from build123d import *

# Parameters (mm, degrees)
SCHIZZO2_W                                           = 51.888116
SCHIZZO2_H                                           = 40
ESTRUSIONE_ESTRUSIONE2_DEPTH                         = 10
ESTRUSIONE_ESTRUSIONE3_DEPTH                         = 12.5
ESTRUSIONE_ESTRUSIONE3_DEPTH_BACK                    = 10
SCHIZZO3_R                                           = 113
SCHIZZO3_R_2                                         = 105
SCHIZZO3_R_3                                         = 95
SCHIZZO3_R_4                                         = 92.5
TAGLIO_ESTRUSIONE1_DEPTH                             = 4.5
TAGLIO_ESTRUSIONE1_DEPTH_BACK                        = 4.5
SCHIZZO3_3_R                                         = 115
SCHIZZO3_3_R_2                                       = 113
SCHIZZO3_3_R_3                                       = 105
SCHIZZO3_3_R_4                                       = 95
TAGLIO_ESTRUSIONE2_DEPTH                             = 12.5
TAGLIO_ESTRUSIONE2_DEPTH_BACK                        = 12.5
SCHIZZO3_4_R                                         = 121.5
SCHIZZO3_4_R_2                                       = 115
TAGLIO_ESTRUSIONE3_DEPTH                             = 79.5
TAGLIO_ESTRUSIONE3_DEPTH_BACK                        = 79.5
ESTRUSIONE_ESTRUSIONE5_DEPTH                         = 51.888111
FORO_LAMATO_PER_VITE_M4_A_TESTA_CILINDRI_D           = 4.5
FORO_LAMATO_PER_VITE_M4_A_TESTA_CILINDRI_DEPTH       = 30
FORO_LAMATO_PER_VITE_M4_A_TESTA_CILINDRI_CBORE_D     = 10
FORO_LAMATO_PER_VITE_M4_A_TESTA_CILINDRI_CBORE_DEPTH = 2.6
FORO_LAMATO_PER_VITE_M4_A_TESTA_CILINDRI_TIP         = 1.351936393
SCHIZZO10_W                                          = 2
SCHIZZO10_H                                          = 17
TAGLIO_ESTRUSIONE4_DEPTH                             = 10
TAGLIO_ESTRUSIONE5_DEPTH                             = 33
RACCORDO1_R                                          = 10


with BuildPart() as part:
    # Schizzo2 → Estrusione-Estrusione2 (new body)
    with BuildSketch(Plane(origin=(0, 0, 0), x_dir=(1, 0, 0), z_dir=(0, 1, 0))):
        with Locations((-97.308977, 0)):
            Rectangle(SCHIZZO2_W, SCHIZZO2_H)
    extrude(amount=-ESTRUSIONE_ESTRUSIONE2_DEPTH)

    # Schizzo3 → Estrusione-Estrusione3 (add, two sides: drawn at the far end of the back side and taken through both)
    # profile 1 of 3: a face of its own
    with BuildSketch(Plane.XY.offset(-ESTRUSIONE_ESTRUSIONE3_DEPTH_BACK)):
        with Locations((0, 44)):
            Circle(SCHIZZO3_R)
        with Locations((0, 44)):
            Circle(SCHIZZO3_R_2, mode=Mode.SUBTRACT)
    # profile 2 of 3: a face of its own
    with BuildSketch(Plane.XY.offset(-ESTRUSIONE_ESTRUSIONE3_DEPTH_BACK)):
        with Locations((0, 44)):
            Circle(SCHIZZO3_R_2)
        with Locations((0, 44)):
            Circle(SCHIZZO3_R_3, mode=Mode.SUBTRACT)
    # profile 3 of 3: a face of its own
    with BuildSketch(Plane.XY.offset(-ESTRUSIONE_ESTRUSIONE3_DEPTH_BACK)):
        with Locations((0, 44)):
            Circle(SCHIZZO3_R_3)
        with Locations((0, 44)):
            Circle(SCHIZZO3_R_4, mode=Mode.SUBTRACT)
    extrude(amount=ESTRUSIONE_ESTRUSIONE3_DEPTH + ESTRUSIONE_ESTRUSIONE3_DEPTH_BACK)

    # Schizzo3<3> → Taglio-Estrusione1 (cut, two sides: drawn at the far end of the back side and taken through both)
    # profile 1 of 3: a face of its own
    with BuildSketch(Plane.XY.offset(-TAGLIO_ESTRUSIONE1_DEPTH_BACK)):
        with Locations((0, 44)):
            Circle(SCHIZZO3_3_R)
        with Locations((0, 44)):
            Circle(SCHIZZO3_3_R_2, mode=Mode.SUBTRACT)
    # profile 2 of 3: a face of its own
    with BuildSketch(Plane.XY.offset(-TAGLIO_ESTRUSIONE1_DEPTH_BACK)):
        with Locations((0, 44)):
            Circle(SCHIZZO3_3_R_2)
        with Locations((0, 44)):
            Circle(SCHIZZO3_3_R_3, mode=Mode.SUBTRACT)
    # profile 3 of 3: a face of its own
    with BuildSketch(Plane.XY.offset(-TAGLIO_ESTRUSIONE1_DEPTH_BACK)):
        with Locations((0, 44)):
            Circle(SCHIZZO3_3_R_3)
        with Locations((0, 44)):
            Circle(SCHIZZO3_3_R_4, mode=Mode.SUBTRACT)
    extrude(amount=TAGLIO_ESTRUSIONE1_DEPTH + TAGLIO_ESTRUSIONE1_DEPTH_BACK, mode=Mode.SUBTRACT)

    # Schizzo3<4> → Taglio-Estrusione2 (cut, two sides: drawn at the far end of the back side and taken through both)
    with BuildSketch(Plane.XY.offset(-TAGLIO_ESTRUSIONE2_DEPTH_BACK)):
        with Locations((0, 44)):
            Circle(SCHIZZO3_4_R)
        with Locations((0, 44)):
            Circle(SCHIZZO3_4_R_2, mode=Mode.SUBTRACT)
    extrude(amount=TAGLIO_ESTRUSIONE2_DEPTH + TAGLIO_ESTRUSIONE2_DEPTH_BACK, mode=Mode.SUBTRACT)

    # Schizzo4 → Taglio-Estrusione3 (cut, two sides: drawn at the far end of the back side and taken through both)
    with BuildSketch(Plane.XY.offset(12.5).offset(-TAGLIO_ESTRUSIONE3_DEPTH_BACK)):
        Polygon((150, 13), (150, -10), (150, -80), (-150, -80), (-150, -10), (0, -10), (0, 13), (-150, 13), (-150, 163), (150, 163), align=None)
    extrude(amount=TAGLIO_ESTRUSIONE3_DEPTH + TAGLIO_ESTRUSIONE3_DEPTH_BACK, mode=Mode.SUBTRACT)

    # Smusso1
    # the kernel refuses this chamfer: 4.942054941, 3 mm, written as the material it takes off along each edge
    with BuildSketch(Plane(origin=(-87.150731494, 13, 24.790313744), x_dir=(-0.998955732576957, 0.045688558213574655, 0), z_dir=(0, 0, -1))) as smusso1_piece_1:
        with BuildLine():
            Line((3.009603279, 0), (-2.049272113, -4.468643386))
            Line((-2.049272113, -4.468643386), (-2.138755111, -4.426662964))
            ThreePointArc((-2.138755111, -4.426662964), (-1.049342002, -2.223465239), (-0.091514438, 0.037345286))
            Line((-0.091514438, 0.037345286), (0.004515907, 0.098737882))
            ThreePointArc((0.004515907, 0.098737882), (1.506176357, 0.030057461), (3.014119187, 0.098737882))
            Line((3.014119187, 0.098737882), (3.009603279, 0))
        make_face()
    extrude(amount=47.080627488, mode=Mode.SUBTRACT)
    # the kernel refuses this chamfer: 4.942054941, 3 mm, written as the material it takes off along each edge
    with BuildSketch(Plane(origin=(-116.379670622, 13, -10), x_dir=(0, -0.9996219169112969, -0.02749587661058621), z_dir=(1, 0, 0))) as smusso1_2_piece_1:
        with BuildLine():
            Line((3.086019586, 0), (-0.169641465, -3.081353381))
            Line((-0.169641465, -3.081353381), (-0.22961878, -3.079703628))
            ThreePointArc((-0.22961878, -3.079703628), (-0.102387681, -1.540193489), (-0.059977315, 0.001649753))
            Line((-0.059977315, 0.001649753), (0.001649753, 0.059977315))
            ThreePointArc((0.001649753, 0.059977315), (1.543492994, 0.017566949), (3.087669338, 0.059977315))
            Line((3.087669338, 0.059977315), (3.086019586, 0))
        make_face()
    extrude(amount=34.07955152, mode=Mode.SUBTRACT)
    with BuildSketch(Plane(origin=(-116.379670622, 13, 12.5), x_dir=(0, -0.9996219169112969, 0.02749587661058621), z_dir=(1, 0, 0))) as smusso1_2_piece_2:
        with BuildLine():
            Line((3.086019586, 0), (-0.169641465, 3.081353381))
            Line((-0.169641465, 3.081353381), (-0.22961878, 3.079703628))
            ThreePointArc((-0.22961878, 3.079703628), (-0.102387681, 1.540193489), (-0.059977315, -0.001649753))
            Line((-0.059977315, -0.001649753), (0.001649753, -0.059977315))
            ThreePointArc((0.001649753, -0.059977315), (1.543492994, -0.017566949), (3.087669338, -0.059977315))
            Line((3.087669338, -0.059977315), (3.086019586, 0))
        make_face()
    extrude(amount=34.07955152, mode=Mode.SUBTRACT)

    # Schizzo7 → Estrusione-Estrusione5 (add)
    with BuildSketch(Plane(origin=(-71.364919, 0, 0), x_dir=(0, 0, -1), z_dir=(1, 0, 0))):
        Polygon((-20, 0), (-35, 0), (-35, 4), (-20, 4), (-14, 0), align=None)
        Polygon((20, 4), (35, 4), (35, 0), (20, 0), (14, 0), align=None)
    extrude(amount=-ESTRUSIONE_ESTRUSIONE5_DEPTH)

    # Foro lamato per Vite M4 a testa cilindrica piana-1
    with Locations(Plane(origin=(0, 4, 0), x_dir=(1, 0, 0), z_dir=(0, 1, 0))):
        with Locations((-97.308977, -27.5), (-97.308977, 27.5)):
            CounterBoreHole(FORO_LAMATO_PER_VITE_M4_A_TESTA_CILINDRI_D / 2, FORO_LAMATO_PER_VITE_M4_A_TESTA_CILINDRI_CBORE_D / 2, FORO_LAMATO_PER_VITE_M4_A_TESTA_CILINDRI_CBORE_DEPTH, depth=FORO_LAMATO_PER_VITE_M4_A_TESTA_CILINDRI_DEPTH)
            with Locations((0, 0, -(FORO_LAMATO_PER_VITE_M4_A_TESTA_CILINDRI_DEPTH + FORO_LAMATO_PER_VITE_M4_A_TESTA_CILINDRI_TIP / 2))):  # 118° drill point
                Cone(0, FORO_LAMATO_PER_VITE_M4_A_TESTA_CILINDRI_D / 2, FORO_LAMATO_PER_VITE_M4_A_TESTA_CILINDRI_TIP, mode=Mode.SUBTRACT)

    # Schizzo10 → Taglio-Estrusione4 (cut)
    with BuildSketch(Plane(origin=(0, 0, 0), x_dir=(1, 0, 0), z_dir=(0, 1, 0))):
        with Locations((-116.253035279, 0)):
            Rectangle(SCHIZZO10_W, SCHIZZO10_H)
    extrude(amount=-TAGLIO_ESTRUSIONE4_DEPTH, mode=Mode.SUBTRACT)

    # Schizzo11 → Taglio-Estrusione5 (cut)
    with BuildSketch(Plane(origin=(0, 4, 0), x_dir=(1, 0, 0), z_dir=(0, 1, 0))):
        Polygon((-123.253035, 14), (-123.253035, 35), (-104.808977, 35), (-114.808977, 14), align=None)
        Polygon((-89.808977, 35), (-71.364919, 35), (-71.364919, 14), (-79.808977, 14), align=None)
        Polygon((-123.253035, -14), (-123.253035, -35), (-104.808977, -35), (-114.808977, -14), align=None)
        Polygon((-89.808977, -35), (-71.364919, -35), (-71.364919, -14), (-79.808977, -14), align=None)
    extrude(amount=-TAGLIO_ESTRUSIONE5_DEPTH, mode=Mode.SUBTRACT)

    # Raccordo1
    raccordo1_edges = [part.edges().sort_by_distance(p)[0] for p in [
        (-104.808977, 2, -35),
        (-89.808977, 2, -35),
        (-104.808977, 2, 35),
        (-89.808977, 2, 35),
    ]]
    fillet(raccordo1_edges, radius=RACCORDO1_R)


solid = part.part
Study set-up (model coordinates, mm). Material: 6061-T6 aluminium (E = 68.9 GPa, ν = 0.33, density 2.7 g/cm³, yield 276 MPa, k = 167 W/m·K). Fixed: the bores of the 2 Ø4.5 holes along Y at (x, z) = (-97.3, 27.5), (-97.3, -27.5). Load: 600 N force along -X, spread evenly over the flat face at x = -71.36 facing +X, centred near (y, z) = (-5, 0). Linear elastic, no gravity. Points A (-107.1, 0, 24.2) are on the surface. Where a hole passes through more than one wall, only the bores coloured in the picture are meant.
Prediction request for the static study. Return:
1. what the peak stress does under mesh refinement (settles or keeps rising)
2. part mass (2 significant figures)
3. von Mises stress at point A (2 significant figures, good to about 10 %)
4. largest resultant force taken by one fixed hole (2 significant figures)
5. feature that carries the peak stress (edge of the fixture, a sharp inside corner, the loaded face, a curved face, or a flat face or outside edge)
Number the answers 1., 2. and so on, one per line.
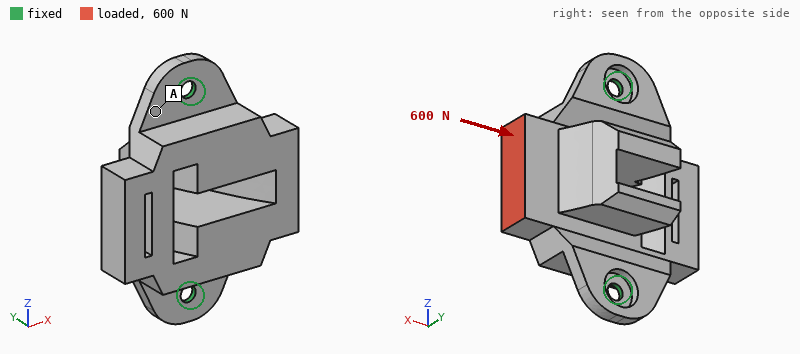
1. keeps rising
2. 57 g
3. 12 MPa
4. 320 N
5. edge of the fixture
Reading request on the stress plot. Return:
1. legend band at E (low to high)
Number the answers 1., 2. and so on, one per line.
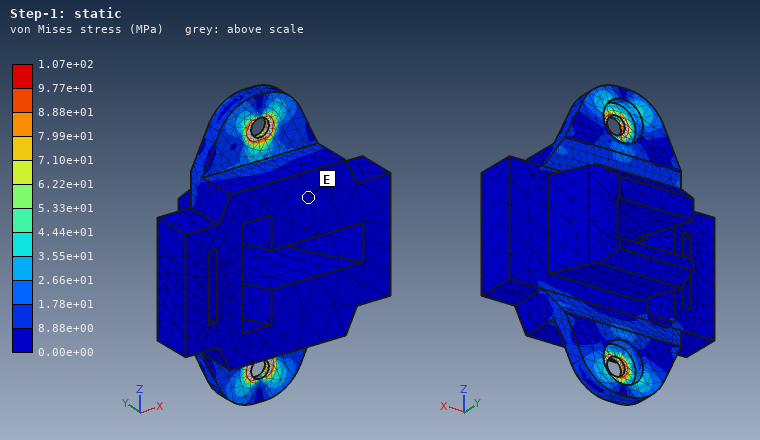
1. 0.00e+00 to 8.88e+00 MPa
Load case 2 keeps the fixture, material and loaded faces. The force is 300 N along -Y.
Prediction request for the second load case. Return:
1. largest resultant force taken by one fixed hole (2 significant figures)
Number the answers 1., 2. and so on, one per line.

1. 160 N
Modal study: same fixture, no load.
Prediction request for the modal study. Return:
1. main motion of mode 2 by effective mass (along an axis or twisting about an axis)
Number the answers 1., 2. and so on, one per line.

1. along Y
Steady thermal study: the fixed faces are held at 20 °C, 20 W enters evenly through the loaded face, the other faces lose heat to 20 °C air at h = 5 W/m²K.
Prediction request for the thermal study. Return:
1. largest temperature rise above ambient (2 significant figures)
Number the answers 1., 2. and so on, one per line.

1. 23 K
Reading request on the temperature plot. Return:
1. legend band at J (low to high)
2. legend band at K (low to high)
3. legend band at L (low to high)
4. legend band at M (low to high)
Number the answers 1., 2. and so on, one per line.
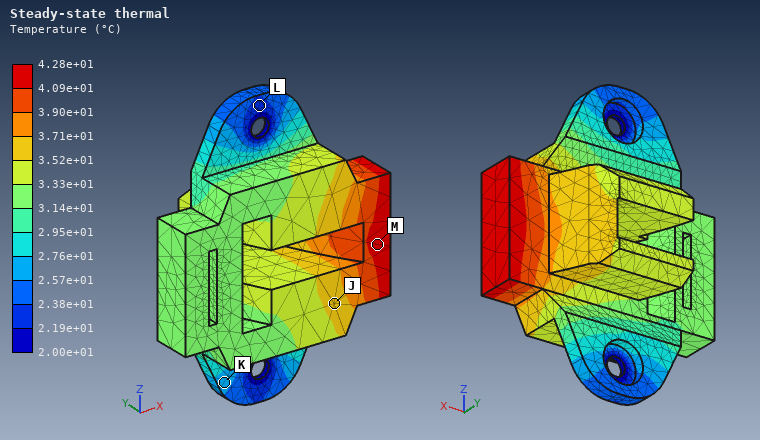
1. 3.52e+01 to 3.71e+01 °C
2. 2.57e+01 to 2.76e+01 °C
3. 2.19e+01 to 2.38e+01 °C
4. 4.09e+01 to 4.28e+01 °C
